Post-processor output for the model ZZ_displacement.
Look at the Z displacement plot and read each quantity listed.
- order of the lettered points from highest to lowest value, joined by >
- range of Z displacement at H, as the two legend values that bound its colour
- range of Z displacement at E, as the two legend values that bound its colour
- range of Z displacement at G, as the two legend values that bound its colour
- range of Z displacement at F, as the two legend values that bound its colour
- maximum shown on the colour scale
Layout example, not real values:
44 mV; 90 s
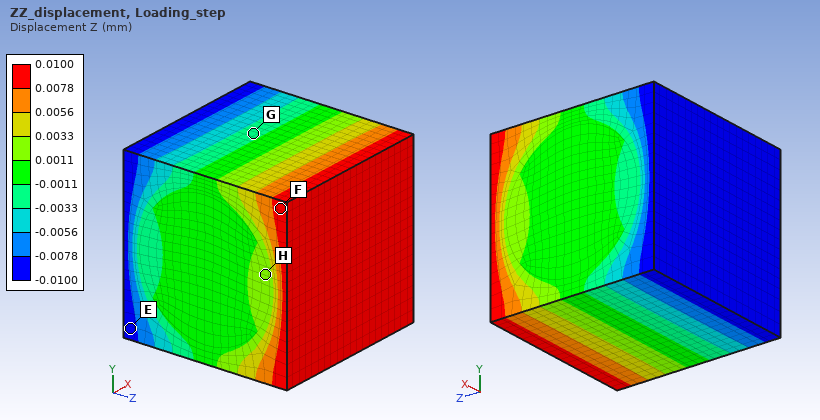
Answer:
F > H > G > E; 0.0011 to 0.0033 mm; -0.0100 to -0.0078 mm; -0.0033 to -0.0011 mm; 0.0078 to 0.0100 mm; 0.0100 mm
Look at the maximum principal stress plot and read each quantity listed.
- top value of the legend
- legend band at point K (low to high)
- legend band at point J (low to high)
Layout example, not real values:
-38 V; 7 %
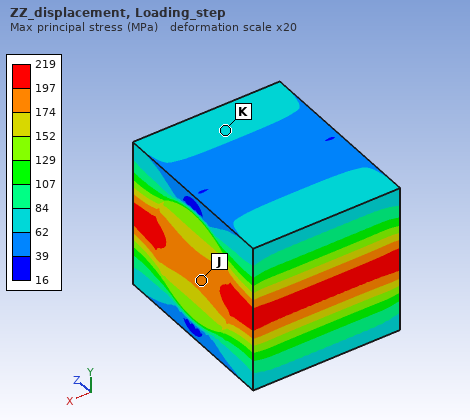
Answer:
219 MPa; 62 to 84 MPa; 174 to 197 MPa
